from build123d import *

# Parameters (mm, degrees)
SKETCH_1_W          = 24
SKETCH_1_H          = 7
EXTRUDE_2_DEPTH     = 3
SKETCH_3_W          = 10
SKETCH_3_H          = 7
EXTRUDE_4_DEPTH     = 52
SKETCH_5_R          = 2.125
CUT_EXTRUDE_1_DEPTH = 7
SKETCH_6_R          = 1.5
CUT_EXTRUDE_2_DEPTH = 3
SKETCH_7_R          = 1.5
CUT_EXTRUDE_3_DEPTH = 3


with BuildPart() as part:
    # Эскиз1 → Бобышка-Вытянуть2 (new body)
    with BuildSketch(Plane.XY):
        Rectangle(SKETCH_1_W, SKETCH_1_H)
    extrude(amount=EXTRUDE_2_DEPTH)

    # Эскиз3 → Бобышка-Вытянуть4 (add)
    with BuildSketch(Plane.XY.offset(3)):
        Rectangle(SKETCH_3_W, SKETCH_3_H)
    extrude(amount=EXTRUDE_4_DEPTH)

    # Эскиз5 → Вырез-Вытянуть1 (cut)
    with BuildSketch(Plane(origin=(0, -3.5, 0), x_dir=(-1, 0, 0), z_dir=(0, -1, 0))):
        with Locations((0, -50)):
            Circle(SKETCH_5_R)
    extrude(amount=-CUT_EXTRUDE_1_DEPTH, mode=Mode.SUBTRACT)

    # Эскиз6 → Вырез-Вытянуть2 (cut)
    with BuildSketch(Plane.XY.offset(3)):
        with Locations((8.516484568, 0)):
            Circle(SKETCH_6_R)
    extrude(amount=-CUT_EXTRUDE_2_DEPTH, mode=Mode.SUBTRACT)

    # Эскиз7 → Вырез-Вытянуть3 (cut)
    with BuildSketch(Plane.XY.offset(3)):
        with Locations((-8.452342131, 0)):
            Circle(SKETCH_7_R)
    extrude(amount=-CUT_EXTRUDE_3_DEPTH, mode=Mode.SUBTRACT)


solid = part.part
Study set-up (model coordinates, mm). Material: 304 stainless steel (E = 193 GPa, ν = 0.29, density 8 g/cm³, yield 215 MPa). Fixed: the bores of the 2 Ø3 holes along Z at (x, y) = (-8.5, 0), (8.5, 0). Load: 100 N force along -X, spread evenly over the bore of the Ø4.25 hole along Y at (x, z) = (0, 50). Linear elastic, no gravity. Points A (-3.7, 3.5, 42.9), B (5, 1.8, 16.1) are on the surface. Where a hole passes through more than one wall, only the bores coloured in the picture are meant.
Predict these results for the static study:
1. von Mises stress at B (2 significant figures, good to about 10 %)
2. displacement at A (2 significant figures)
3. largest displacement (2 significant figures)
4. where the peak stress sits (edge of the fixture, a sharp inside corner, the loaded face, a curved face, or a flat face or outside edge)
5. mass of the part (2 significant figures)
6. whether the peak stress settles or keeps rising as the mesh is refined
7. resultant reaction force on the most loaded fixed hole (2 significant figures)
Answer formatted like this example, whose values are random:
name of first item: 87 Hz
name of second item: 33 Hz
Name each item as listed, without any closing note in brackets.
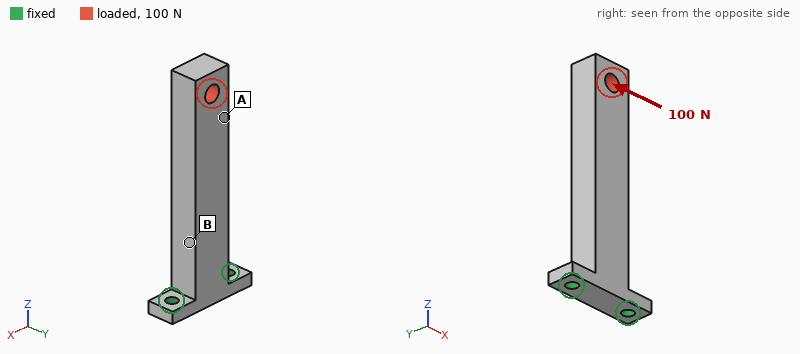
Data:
von Mises stress at B: 29 MPa
displacement at A: 37 µm
largest displacement: 53 µm
where the peak stress sits: edge of the fixture
mass of the part: 32 g
whether the peak stress settles or keeps rising as the mesh is refined: keeps rising
resultant reaction force on the most loaded fixed hole: 390 N
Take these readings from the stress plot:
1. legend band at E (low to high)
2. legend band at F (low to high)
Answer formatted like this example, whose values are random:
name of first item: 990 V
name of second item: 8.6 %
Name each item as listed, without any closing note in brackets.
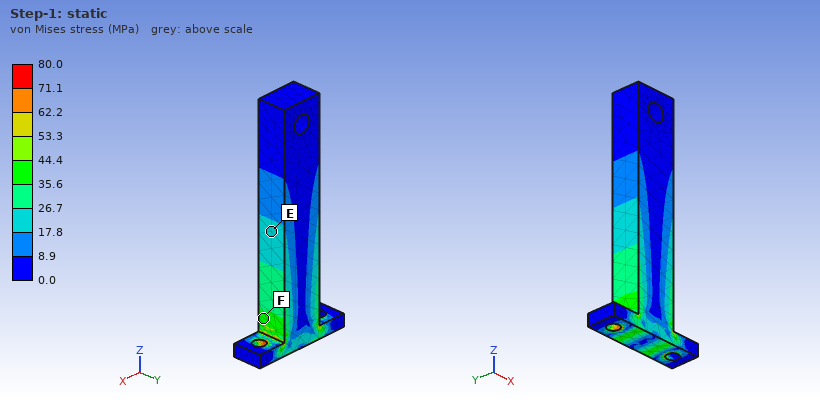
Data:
legend band at E: 17.8 to 26.7 MPa
legend band at F: 35.6 to 44.4 MPa
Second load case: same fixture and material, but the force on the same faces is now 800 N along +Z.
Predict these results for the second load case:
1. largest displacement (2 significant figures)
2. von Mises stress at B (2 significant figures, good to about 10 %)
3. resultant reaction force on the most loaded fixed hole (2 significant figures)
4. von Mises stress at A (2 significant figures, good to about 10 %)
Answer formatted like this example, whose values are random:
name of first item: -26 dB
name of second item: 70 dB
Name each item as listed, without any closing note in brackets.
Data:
largest displacement: 5.2 µm
von Mises stress at B: 11 MPa
resultant reaction force on the most loaded fixed hole: 430 N
von Mises stress at A: 12 MPa
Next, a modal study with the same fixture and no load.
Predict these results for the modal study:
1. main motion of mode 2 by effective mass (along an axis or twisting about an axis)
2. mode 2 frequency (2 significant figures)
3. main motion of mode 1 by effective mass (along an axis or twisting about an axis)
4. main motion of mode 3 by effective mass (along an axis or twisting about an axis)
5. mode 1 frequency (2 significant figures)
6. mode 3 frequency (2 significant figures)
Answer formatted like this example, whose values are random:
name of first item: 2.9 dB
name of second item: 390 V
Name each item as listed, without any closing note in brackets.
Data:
main motion of mode 2 by effective mass: along X
mode 2 frequency: 2400 Hz
main motion of mode 1 by effective mass: along Y
main motion of mode 3 by effective mass: along Y
mode 1 frequency: 1200 Hz
mode 3 frequency: 9000 Hz
